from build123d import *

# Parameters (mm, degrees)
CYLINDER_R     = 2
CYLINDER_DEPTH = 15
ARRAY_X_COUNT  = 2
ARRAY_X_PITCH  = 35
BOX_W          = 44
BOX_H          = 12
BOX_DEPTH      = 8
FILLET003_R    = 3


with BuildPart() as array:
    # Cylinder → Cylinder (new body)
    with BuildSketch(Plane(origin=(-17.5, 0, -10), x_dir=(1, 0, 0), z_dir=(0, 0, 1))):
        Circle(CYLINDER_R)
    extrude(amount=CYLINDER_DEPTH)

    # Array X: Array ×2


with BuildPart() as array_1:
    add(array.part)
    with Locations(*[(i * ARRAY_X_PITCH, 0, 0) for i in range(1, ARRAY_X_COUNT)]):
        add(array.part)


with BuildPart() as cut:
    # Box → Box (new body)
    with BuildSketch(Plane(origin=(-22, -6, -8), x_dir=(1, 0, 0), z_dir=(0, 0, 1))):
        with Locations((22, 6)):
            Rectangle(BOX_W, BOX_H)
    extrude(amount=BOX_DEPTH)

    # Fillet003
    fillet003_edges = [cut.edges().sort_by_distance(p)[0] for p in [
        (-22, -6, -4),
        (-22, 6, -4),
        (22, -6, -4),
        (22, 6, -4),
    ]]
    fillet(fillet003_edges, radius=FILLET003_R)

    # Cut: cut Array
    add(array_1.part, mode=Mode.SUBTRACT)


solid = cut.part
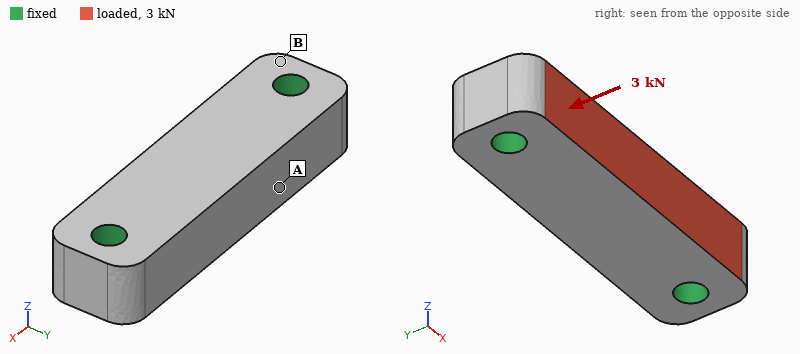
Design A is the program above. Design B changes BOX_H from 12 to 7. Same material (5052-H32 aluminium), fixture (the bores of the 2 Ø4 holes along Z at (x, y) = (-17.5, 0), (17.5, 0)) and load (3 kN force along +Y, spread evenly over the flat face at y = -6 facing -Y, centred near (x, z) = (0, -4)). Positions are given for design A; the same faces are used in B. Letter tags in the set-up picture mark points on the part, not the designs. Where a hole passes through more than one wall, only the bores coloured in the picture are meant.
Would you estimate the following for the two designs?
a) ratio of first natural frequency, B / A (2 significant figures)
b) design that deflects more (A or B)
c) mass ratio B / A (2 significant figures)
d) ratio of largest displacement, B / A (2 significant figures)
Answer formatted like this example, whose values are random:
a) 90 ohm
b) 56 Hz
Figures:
a) 0.92
b) B
c) 0.56
d) 2.3
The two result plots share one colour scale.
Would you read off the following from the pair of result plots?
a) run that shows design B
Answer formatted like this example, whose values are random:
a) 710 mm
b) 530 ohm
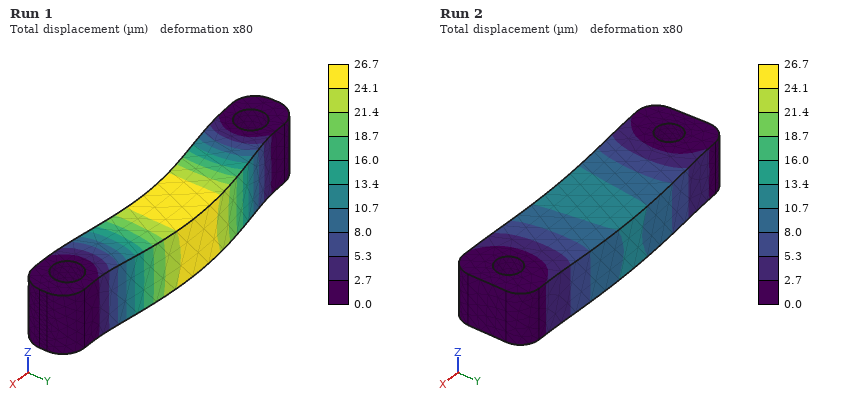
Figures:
a) Run 1
